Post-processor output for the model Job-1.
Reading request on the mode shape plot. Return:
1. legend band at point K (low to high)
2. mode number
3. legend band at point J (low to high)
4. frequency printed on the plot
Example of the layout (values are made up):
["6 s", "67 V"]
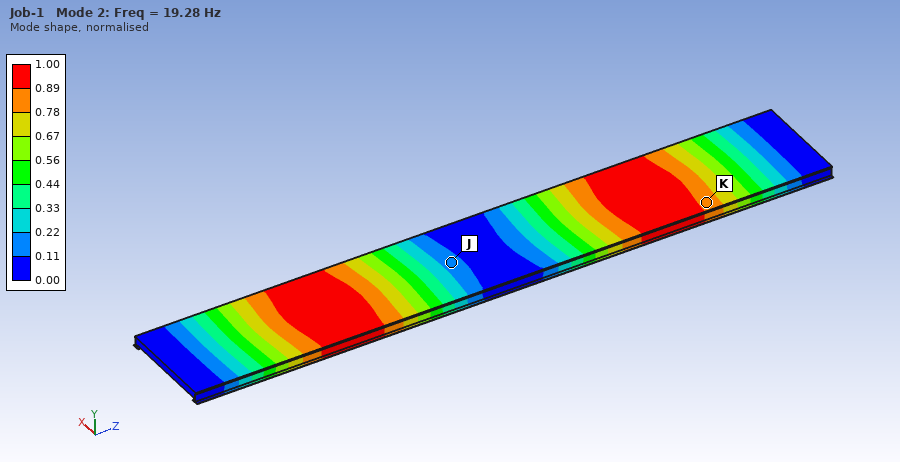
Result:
["0.78 to 0.89", "2", "0.11 to 0.22", "19.28 Hz"]
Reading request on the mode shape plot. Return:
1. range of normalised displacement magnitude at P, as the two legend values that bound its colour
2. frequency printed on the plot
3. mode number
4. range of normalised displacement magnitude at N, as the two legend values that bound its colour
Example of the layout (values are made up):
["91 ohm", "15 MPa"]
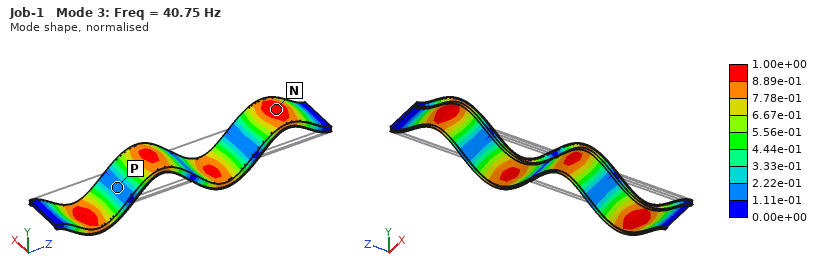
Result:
["1.11e-01 to 2.22e-01", "40.75 Hz", "3", "8.89e-01 to 1.00e+00"]
